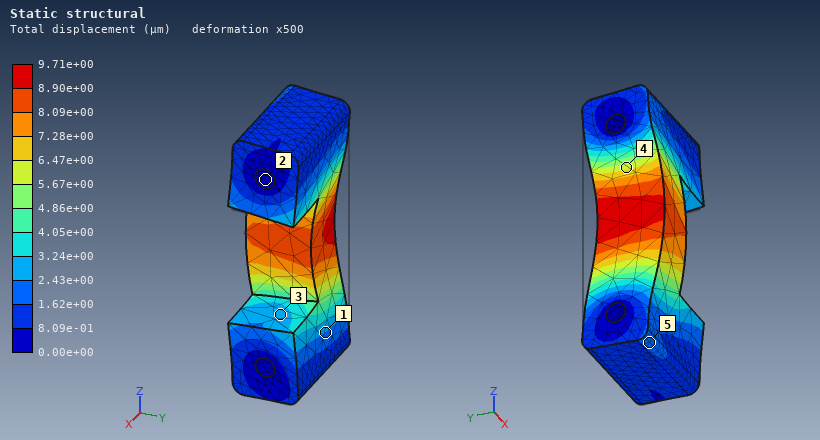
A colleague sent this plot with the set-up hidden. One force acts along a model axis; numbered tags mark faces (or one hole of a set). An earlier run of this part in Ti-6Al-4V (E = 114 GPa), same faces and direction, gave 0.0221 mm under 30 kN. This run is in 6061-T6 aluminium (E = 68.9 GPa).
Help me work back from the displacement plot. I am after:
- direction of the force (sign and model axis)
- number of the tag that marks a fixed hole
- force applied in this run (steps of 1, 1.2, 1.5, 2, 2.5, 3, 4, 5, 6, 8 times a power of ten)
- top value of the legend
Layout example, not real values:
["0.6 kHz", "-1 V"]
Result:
["-Y", "2", "8 kN", "9.71e+00 µm"]
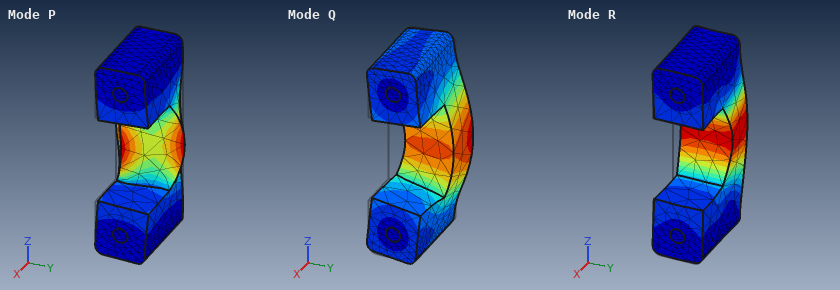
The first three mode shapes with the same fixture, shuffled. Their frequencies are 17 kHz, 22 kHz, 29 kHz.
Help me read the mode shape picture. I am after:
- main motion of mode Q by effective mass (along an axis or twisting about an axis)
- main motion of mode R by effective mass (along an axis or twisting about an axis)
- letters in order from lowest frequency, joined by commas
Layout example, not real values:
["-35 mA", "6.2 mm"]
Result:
["along Y", "along X", "Q, R, P"]
